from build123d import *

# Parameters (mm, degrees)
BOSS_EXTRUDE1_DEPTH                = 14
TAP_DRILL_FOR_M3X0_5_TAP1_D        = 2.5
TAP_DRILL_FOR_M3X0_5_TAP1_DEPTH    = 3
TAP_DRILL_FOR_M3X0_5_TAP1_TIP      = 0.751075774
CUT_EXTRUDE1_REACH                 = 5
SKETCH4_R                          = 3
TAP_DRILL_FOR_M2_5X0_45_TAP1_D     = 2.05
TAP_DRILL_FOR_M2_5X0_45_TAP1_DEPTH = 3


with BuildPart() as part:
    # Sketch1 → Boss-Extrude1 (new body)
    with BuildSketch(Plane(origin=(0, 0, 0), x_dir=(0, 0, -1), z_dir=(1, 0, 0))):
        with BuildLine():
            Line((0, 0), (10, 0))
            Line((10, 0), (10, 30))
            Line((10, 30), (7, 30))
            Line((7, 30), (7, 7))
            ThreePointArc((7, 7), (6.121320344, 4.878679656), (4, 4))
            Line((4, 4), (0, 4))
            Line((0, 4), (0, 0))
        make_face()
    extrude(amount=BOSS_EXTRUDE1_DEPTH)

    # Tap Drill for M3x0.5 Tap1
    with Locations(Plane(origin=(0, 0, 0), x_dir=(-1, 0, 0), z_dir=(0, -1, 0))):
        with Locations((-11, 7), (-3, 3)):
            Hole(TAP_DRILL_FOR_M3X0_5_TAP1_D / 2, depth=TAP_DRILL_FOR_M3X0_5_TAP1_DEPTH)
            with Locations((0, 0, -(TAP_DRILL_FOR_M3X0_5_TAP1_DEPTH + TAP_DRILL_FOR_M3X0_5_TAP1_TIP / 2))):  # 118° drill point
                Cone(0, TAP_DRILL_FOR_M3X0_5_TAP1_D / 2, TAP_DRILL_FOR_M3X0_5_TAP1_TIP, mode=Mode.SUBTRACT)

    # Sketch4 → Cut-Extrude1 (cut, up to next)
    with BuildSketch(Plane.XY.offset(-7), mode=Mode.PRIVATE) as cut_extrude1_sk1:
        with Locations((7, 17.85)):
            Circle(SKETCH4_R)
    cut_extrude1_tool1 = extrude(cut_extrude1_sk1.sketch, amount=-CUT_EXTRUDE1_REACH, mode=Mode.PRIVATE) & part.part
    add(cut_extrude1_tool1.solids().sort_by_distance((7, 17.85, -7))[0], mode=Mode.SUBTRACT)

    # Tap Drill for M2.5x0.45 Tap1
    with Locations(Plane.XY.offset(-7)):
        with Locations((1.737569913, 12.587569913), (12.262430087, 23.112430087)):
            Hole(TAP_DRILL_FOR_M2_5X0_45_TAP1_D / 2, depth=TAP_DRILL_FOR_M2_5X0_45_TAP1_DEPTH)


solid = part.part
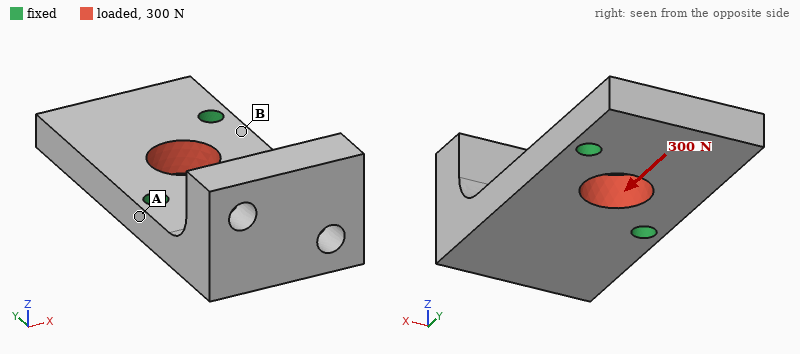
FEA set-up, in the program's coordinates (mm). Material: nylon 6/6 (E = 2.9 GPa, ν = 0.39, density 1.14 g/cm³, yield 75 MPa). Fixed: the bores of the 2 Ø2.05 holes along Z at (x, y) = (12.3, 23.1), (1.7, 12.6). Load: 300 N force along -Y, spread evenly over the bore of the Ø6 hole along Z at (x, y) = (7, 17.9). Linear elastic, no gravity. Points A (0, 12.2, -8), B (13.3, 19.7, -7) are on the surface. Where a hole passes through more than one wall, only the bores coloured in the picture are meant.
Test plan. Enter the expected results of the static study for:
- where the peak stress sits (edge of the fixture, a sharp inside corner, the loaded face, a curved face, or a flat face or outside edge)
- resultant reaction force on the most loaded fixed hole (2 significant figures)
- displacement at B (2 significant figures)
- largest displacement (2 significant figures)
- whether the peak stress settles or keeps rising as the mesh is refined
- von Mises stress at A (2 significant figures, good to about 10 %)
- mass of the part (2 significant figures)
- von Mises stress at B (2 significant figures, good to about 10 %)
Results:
edge of the fixture
150 N
7.4 µm
33 µm
keeps rising
2.9 MPa
1.8 g
7.4 MPa
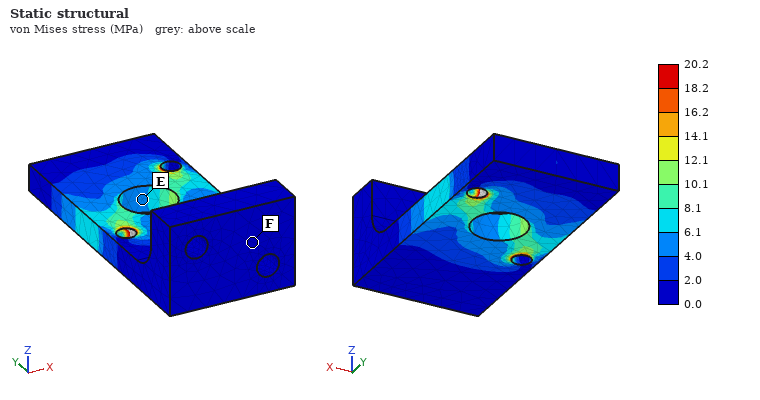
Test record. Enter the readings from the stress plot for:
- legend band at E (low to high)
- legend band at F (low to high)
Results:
4.0 to 6.1 MPa
0.0 to 2.0 MPa
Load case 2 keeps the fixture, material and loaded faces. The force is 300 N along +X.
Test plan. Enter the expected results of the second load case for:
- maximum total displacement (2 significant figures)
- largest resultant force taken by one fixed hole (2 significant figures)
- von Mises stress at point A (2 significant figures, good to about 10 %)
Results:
31 µm
150 N
4.4 MPa
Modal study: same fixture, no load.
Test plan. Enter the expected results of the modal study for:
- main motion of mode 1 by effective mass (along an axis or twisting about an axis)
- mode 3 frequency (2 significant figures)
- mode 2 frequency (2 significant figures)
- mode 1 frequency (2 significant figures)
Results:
along Z
5600 Hz
3700 Hz
1900 Hz
